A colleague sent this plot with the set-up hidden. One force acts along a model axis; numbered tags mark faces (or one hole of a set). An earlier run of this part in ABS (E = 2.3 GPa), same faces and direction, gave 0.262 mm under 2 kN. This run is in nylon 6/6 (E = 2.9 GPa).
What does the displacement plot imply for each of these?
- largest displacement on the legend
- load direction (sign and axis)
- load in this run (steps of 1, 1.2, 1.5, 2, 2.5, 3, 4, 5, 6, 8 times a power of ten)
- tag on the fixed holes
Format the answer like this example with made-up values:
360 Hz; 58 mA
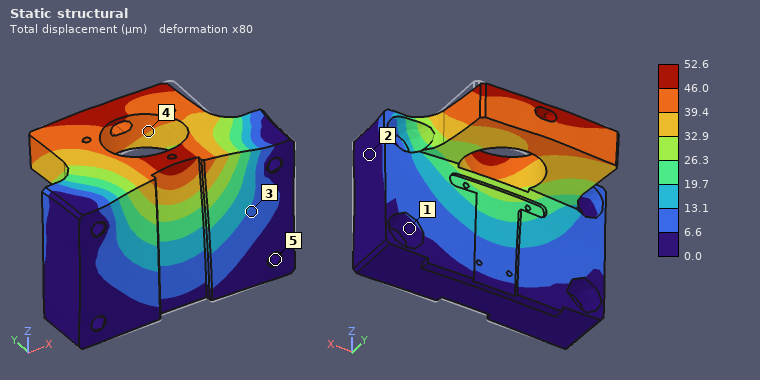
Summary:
52.6 µm; +Y; 500 N; 5
